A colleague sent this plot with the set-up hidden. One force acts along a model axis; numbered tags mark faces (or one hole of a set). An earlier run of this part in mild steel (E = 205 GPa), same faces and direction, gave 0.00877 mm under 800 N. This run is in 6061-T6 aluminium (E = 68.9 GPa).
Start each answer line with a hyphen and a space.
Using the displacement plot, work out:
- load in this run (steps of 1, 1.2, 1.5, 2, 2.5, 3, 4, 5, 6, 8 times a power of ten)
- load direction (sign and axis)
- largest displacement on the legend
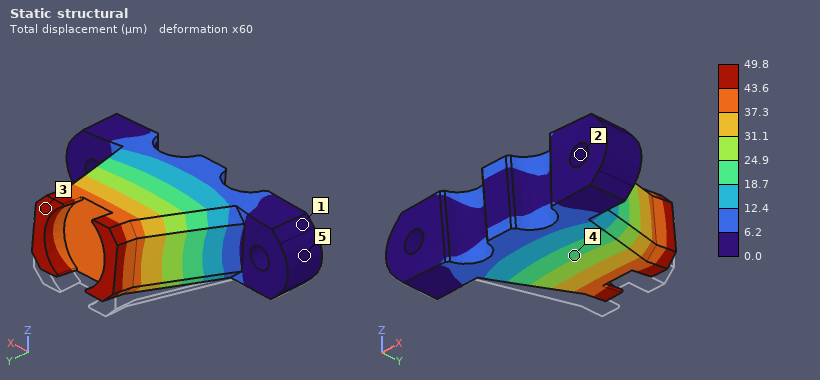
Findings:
- 1.5 kN
- +Z
- 49.8 µm
